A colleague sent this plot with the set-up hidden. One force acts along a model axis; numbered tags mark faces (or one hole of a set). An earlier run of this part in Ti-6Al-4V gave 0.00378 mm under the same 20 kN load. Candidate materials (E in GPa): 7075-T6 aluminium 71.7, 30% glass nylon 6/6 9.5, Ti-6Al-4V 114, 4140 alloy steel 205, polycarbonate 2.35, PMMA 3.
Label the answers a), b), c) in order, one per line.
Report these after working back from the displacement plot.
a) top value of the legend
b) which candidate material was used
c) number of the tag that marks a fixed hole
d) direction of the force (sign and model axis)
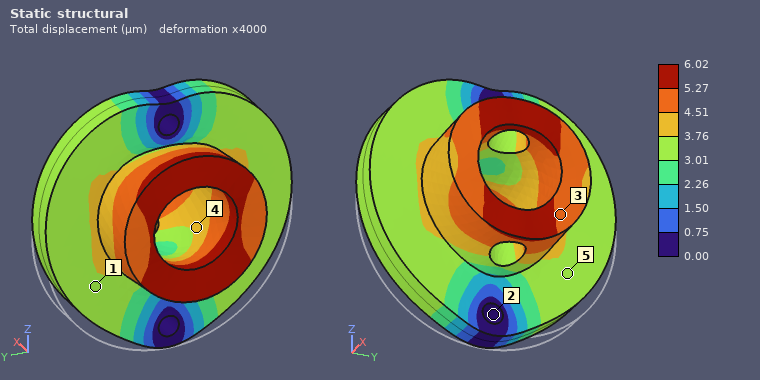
a) 6.02 µm
b) 7075-T6 aluminium
c) 2
d) +Z
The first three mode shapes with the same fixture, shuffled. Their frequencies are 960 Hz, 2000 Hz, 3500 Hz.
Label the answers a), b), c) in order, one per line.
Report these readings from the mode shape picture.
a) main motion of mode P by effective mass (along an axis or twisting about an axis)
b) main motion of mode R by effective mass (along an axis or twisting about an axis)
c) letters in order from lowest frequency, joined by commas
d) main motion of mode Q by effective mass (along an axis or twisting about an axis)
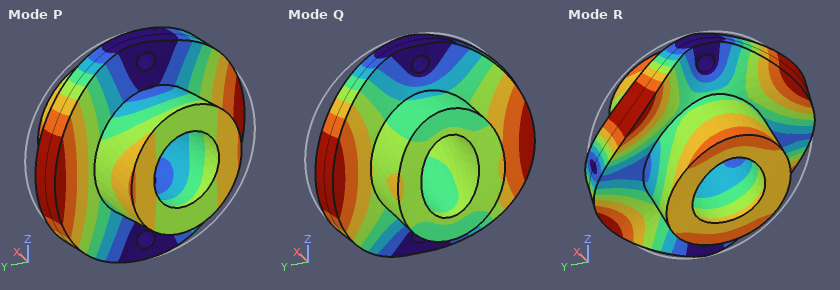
a) twisting about Z
b) twisting about Y
c) P, Q, R
d) along X
